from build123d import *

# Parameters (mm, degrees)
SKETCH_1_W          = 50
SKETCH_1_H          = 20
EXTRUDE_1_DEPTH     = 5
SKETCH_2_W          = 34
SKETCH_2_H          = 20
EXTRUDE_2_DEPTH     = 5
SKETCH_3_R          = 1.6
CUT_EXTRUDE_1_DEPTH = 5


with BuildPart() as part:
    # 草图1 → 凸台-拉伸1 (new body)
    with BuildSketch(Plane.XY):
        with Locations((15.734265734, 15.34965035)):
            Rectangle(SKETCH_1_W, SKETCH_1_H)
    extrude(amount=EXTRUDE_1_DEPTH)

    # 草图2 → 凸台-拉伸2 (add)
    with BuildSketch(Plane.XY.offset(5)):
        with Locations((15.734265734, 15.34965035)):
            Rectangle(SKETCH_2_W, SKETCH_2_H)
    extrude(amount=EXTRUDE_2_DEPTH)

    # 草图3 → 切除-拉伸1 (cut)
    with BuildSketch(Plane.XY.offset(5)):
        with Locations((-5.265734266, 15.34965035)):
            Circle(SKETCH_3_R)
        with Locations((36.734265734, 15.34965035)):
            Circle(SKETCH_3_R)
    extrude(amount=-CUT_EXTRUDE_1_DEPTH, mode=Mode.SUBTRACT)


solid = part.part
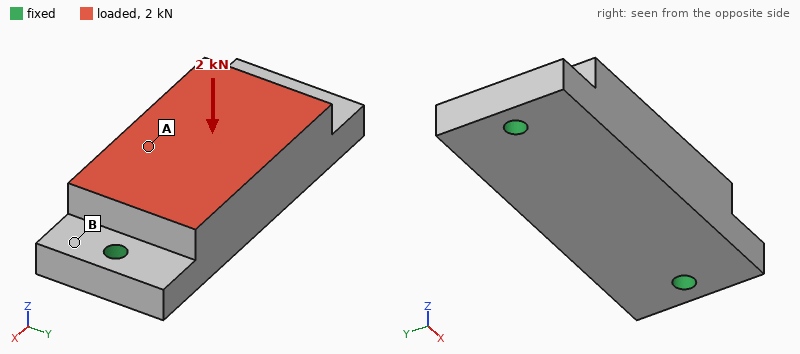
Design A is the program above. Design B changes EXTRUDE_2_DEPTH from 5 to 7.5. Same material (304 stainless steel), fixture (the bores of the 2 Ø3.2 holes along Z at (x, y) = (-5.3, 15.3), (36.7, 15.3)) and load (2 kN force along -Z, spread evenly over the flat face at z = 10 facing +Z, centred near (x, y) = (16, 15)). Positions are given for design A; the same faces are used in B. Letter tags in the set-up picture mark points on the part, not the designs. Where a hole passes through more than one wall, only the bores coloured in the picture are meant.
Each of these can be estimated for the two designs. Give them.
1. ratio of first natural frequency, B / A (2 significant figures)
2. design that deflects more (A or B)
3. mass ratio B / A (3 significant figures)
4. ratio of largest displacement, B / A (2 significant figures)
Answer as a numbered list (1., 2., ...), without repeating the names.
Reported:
1. 0.81
2. A
3. 1.20
4. 0.72
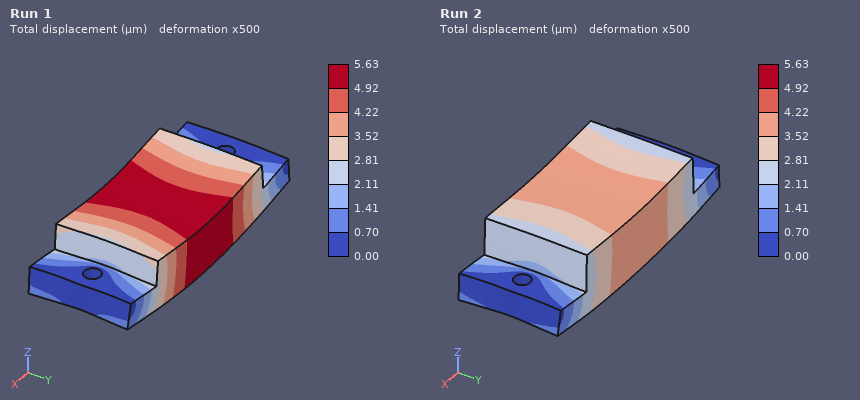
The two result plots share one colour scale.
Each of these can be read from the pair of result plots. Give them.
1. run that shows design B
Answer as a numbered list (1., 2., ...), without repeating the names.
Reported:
1. Run 2
